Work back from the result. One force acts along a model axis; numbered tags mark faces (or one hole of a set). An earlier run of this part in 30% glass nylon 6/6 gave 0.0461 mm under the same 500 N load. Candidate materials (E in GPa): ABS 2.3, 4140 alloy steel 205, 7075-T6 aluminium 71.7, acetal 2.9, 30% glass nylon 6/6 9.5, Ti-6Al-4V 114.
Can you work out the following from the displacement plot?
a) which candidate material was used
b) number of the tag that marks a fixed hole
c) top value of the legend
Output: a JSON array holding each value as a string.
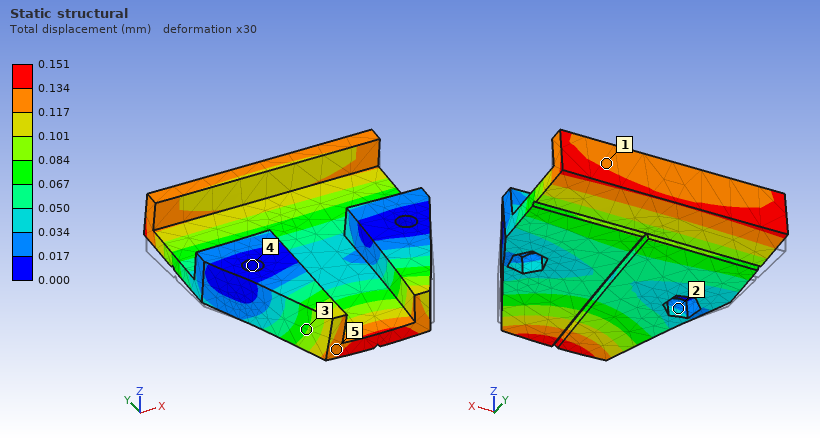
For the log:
["acetal", "4", "0.151 mm"]
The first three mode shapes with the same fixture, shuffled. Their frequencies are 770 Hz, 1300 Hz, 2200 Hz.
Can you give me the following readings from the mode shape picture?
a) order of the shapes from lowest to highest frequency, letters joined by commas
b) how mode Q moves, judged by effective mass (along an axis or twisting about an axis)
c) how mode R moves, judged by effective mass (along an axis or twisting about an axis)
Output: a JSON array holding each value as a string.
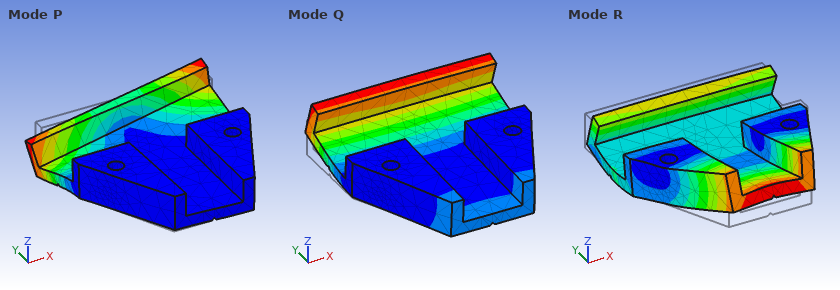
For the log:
["Q, P, R", "along Z", "along Y"]
